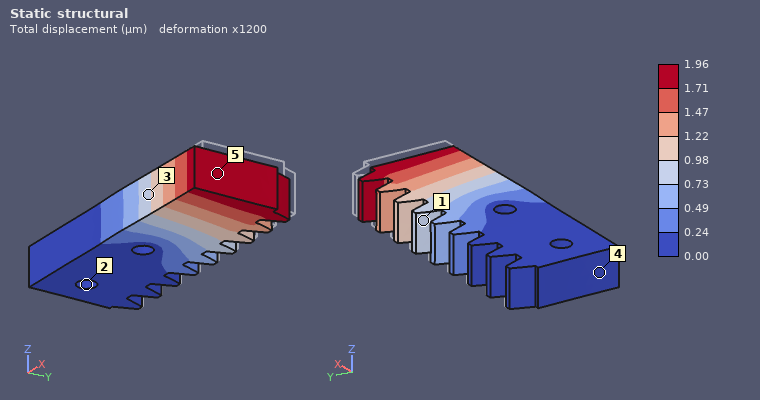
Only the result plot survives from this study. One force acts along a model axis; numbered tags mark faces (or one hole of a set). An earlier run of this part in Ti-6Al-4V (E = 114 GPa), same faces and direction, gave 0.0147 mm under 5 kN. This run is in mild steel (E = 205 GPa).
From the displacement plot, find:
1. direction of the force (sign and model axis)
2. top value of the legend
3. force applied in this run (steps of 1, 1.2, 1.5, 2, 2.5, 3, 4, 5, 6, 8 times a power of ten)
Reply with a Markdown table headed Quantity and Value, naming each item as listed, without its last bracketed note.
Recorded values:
| Quantity | Value |
|---|---|
| direction of the force | -X |
| top value of the legend | 1.96 µm |
| force applied in this run | 1.2 kN |
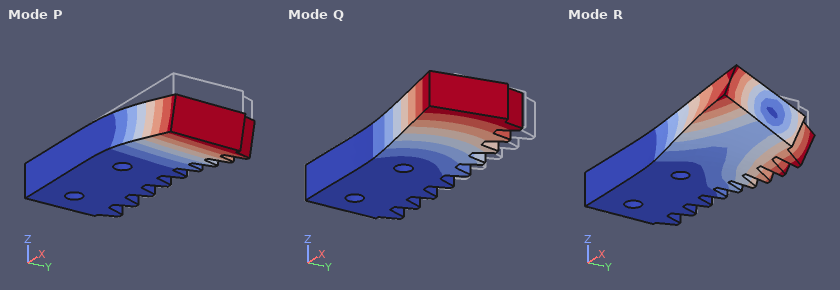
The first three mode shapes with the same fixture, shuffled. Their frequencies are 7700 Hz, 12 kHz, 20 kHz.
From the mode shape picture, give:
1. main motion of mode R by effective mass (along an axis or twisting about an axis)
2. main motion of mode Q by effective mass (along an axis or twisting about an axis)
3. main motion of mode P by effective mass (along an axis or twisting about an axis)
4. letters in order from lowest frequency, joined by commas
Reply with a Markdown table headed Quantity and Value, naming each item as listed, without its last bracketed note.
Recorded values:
| Quantity | Value |
|---|---|
| main motion of mode R by effective mass | twisting about X |
| main motion of mode Q by effective mass | along Y |
| main motion of mode P by effective mass | along Z |
| letters in order from lowest frequency, joined by commas | P, Q, R |
